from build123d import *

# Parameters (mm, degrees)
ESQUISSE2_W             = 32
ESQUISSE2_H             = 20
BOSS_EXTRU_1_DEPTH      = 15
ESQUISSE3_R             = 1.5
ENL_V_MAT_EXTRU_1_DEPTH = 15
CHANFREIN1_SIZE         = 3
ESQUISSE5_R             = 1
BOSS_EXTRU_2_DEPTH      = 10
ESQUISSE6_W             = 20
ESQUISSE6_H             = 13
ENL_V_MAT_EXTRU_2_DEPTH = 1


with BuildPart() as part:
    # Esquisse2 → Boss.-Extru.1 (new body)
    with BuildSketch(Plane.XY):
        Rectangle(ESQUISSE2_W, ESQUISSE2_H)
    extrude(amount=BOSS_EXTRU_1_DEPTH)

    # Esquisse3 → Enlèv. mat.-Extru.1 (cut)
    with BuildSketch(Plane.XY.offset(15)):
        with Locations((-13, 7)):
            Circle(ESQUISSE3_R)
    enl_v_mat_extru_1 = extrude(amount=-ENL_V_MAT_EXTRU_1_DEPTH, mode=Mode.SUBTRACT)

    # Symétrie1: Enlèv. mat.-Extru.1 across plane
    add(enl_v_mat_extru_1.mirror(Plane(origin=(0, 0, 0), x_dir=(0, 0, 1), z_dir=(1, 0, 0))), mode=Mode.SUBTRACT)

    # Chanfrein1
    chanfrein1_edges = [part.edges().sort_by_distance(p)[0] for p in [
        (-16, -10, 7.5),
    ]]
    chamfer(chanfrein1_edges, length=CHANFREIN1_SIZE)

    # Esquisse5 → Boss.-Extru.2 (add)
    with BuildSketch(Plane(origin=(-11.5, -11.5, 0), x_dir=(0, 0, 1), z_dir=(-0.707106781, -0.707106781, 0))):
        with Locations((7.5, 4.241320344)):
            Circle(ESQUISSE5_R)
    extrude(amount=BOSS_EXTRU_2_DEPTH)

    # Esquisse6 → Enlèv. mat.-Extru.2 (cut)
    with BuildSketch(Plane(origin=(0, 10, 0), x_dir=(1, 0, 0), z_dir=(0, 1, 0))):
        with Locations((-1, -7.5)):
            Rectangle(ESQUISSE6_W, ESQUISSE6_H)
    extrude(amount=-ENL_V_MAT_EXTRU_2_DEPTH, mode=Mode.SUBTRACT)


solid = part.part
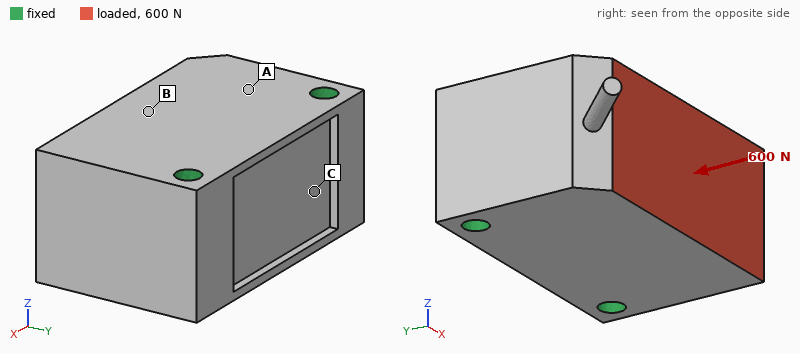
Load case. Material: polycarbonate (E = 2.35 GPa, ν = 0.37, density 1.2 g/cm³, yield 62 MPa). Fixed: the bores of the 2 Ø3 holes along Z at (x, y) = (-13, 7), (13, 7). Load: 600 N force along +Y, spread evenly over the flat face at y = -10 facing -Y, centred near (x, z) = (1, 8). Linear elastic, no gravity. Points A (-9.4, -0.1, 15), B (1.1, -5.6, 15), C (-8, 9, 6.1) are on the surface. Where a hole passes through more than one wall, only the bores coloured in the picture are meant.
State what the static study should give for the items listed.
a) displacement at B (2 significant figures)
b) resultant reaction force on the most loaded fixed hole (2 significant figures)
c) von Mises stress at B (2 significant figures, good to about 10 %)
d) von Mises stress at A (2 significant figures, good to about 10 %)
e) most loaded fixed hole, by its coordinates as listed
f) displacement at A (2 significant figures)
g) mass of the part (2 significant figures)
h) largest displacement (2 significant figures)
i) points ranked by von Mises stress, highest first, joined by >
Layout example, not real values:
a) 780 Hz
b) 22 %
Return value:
a) 16 µm
b) 350 N
c) 1.1 MPa
d) 1.9 MPa
e) (13, 7)
f) 8.0 µm
g) 11 g
h) 17 µm
i) A > B > C
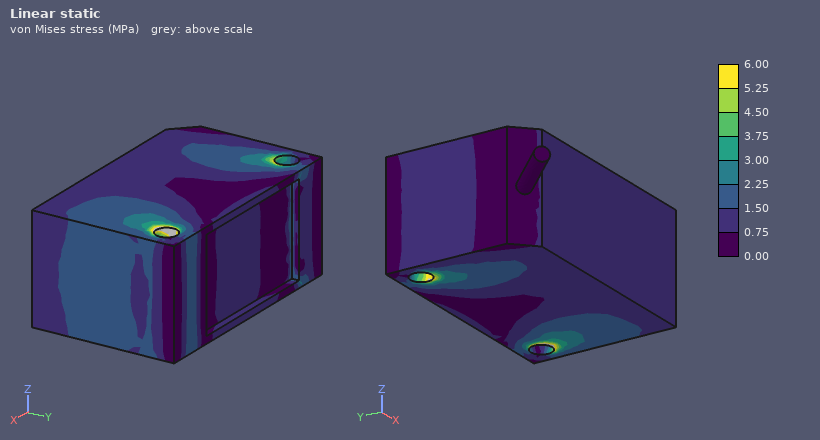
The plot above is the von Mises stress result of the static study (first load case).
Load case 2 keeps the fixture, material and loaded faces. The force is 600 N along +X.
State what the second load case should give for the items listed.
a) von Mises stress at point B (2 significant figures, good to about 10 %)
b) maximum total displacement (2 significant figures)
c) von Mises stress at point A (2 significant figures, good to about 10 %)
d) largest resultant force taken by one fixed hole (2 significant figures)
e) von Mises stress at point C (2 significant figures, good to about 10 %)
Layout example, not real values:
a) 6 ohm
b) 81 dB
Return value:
a) 3.4 MPa
b) 57 µm
c) 2.8 MPa
d) 480 N
e) 1.2 MPa
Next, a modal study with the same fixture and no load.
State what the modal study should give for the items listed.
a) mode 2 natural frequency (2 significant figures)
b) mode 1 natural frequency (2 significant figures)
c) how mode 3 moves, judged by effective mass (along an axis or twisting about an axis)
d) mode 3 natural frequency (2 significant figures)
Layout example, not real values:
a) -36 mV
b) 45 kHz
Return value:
a) 3600 Hz
b) 3500 Hz
c) along Z
d) 5900 Hz
